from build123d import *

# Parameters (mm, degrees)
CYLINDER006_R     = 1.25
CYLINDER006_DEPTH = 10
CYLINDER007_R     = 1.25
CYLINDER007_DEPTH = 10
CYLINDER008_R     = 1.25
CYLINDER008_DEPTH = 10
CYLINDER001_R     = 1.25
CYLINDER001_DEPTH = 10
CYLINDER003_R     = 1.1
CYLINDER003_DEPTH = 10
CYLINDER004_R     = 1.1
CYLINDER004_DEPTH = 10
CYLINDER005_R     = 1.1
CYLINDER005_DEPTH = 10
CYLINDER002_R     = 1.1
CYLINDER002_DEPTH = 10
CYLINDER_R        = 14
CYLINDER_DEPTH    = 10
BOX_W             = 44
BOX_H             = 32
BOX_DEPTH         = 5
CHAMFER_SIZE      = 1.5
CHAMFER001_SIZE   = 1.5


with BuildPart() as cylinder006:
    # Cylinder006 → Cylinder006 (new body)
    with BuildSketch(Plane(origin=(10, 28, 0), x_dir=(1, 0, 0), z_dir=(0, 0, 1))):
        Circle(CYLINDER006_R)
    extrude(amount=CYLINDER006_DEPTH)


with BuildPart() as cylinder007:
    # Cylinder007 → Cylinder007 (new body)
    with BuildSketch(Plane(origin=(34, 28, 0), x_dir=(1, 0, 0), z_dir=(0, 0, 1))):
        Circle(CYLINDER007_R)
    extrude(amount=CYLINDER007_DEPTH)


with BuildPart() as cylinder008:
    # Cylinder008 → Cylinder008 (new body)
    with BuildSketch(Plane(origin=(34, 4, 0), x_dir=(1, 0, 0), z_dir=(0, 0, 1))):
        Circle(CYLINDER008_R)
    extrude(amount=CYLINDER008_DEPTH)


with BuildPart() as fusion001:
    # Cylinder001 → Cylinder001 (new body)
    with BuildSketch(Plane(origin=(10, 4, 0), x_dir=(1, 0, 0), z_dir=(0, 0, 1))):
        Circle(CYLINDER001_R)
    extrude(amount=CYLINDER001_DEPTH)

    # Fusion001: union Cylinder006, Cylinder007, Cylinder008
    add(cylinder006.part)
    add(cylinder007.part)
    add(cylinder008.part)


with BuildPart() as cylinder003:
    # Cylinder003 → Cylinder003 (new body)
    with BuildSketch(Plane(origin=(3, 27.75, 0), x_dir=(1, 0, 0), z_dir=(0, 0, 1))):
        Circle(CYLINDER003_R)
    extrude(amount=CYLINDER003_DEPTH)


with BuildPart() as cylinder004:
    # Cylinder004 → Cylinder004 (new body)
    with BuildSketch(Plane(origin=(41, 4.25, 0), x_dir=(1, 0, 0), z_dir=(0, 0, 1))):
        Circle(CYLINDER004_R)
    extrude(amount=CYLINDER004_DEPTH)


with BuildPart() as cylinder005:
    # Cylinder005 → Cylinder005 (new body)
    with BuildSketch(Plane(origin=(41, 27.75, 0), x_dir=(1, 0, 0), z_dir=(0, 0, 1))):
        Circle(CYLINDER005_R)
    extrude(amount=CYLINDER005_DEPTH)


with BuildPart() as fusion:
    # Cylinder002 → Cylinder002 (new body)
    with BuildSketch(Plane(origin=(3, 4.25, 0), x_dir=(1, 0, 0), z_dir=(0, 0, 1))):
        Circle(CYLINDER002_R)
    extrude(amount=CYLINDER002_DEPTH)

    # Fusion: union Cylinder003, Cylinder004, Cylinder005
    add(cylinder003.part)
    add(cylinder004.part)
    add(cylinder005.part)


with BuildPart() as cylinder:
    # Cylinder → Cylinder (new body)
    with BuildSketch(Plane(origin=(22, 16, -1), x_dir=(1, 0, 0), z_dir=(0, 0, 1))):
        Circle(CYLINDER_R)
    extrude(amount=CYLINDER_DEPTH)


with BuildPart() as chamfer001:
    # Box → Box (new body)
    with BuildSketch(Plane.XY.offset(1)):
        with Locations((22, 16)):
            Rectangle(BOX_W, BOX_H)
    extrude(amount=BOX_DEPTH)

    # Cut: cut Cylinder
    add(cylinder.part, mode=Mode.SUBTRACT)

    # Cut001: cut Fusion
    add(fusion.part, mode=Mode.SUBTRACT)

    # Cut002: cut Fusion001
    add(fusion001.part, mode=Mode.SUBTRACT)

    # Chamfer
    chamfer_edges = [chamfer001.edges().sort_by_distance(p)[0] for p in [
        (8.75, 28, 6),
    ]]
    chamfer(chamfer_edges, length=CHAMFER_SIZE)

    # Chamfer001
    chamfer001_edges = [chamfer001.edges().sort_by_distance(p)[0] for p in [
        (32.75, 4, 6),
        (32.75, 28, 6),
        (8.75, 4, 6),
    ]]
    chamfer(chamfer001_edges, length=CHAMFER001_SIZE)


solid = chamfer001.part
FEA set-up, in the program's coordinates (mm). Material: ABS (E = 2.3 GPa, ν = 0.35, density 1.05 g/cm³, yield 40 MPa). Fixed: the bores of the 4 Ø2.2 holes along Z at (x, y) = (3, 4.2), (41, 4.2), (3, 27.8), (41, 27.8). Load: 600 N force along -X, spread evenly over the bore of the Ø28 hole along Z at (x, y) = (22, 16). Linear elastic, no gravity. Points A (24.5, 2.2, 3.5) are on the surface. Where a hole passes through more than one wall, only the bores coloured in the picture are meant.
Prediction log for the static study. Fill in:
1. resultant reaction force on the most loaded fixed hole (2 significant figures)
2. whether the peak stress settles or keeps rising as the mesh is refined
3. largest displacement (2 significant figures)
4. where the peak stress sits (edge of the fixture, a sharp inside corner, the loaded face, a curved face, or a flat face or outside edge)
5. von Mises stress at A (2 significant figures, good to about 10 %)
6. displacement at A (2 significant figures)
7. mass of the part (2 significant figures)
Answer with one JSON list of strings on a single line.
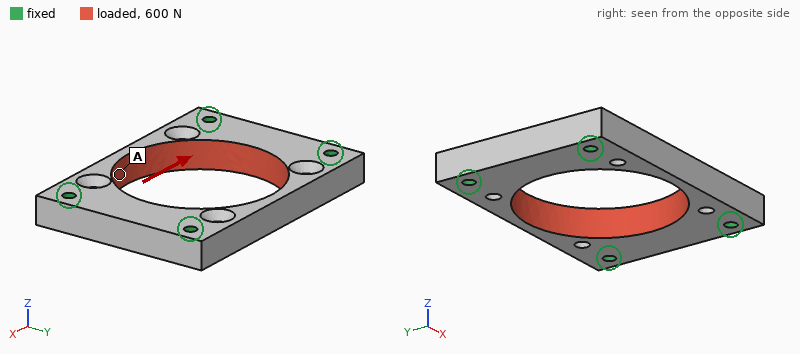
["150 N", "keeps rising", "31 µm", "edge of the fixture", "2.6 MPa", "24 µm", "3.9 g"]
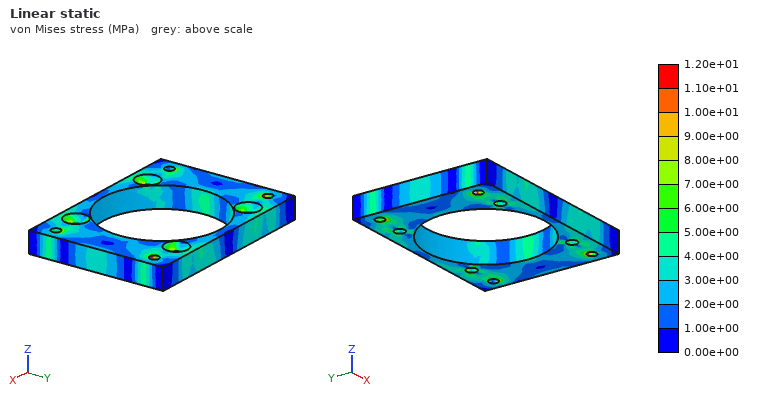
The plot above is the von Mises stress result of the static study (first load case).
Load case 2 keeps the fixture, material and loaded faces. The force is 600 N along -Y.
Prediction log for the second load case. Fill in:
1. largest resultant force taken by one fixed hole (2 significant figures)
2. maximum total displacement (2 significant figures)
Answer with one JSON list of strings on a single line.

["150 N", "0.19 mm"]
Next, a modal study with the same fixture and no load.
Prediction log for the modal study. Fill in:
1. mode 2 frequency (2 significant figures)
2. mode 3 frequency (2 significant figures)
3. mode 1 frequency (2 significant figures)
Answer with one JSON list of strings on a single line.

["6000 Hz", "7800 Hz", "5800 Hz"]
